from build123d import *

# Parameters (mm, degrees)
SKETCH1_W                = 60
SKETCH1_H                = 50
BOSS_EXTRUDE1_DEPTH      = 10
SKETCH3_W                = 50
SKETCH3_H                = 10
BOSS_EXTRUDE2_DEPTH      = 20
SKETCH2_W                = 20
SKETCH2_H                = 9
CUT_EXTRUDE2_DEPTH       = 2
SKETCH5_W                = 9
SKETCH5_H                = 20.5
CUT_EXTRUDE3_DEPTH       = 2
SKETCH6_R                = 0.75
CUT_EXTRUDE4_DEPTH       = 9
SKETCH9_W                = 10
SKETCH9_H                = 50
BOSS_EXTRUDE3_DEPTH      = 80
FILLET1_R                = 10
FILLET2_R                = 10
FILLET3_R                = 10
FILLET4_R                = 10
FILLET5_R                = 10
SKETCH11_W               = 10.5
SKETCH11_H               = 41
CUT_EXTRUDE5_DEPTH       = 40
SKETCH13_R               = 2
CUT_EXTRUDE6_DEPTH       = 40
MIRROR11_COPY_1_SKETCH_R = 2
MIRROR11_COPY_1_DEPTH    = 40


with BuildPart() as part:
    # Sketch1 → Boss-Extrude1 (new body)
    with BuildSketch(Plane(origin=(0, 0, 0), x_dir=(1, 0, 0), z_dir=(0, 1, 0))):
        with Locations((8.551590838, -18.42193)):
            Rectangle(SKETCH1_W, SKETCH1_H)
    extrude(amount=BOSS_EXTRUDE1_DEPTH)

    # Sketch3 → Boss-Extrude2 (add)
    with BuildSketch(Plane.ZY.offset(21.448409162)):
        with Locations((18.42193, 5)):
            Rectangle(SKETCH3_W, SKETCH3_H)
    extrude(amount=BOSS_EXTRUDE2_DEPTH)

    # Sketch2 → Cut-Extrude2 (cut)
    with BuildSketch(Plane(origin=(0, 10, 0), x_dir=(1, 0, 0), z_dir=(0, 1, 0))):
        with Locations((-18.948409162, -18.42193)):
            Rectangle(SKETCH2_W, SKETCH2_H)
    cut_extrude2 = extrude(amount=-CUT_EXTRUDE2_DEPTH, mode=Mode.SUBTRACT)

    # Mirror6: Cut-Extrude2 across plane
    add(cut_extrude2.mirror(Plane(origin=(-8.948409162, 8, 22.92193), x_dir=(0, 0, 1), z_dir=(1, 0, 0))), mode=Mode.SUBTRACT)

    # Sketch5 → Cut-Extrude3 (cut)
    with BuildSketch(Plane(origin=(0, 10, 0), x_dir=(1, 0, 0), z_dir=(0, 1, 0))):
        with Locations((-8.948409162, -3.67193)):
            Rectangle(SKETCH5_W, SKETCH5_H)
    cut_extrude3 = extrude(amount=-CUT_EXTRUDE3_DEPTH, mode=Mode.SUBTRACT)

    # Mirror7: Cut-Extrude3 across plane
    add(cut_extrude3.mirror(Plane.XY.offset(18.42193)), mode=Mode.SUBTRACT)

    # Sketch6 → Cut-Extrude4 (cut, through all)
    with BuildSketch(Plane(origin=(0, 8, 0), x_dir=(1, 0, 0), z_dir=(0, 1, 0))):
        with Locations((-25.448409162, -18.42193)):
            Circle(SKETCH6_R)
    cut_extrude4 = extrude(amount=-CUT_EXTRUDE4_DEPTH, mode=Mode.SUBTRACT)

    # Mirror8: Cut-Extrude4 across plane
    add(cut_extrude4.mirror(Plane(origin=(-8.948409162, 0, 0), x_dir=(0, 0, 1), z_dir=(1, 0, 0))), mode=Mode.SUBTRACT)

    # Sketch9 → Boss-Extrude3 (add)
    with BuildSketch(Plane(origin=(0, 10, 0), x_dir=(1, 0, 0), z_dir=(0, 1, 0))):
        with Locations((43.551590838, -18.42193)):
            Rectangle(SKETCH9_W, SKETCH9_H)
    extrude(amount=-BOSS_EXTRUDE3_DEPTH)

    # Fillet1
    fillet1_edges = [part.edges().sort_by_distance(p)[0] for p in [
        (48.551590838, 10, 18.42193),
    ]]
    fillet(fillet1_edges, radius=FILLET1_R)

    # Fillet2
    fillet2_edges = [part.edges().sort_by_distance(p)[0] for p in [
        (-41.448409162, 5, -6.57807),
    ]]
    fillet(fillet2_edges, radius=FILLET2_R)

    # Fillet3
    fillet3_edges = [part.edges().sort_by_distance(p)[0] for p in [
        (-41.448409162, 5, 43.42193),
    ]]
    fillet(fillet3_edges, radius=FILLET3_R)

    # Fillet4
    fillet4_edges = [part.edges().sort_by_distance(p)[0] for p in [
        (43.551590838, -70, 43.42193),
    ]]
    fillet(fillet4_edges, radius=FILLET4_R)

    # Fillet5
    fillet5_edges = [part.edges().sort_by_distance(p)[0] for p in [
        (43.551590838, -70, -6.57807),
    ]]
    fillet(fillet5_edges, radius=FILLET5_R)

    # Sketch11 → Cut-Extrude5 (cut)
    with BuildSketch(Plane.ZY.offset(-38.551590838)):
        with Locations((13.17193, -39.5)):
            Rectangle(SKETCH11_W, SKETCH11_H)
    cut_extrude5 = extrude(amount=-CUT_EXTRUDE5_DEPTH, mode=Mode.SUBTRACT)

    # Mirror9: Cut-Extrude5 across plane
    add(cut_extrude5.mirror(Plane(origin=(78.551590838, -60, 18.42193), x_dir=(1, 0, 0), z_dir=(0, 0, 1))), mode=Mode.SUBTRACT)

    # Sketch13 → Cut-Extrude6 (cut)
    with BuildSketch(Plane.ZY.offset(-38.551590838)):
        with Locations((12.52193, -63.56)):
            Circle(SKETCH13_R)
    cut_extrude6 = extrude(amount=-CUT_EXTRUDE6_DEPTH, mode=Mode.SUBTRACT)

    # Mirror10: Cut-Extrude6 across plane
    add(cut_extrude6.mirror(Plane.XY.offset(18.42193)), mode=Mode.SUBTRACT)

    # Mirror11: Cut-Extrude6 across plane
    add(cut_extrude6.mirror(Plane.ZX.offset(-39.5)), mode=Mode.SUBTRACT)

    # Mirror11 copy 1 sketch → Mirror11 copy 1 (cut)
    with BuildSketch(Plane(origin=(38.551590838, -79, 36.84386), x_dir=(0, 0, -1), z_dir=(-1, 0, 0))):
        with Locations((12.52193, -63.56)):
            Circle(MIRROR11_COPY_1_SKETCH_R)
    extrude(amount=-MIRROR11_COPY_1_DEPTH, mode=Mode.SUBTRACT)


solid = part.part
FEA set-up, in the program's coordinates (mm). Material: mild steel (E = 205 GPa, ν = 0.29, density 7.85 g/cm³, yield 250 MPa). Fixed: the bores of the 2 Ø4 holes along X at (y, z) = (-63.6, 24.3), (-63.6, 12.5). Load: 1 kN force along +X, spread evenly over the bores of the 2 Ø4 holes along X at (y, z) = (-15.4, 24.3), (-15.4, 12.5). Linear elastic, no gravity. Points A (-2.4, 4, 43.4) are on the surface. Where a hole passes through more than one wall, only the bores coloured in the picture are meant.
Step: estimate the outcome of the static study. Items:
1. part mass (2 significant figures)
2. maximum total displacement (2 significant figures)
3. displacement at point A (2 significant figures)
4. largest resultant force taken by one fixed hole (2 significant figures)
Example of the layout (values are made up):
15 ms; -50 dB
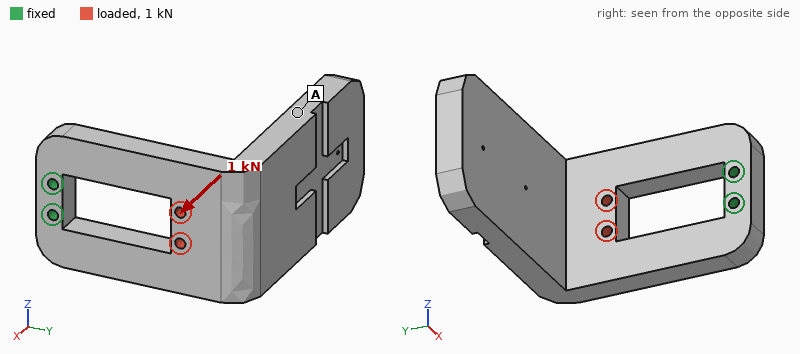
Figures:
530 g; 0.40 mm; 0.28 mm; 500 N
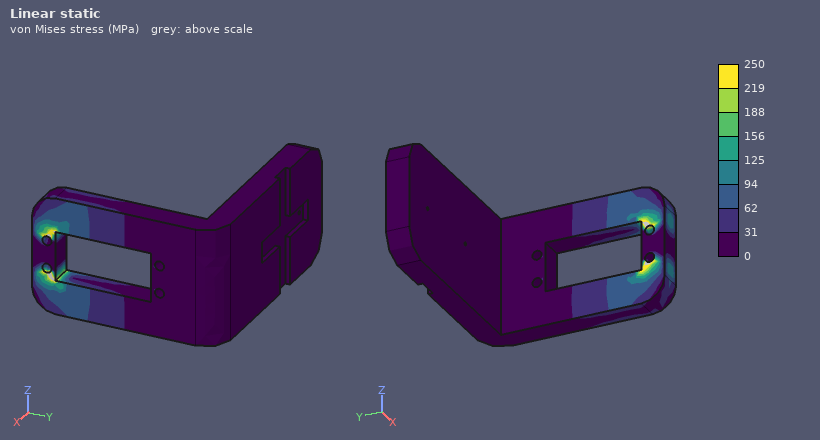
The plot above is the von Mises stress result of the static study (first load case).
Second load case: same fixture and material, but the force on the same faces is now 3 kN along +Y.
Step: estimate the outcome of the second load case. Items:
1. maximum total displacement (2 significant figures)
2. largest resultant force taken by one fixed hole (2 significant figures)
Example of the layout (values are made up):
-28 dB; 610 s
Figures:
8.3 µm; 1.5 kN
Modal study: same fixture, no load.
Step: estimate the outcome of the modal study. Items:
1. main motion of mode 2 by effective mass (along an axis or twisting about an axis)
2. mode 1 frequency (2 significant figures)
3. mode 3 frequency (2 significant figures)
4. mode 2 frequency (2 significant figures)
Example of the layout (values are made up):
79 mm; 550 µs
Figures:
along Z; 320 Hz; 1100 Hz; 490 Hz
